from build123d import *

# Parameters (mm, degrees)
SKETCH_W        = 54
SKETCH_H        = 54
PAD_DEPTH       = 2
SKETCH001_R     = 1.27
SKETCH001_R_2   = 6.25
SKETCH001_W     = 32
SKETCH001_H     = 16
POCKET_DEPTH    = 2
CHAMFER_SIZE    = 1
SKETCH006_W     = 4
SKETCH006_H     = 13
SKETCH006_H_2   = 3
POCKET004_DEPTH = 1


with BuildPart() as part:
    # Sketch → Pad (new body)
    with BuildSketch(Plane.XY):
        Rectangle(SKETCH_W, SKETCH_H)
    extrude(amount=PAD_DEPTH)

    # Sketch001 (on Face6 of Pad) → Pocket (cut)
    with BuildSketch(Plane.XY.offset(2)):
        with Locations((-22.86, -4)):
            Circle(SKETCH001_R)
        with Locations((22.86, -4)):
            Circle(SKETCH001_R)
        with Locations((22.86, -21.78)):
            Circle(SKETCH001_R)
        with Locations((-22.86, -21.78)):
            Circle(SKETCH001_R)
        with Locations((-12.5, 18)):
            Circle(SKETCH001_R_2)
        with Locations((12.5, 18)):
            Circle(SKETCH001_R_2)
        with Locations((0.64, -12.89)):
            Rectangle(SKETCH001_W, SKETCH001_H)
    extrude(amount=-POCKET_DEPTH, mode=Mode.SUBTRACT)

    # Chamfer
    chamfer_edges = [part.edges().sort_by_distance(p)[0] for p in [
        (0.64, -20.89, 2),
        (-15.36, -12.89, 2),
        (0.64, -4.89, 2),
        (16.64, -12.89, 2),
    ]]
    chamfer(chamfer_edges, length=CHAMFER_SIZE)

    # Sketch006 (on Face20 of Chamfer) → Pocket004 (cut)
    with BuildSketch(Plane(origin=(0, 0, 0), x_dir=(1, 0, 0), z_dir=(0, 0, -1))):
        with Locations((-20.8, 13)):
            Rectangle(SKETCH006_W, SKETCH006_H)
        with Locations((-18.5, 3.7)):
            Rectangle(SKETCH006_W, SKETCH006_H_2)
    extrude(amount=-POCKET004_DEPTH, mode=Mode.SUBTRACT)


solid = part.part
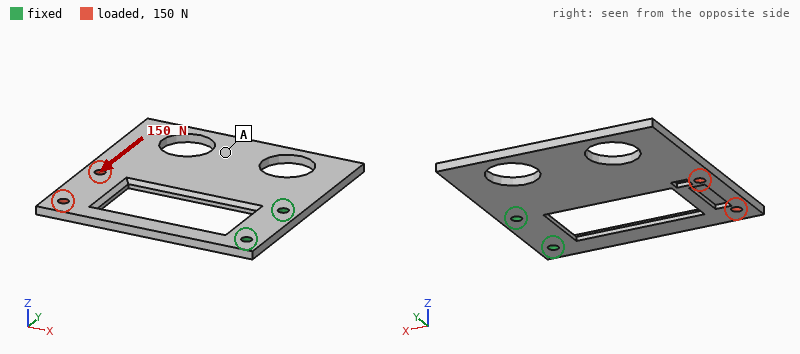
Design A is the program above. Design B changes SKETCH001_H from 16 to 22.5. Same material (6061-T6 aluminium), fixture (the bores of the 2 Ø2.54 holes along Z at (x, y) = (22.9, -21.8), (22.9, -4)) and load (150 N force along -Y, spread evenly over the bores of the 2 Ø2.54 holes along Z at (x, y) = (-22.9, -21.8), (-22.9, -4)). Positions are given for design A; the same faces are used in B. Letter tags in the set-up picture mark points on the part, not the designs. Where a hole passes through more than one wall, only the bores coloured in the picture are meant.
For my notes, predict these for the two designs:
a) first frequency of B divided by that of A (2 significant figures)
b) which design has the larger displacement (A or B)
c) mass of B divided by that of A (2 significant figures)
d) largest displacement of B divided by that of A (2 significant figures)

0.88
B
0.90
1.6
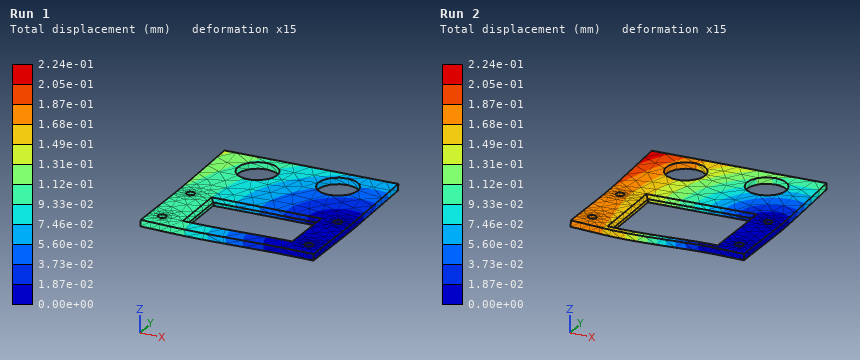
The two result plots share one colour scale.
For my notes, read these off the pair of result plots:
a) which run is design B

Run 2
